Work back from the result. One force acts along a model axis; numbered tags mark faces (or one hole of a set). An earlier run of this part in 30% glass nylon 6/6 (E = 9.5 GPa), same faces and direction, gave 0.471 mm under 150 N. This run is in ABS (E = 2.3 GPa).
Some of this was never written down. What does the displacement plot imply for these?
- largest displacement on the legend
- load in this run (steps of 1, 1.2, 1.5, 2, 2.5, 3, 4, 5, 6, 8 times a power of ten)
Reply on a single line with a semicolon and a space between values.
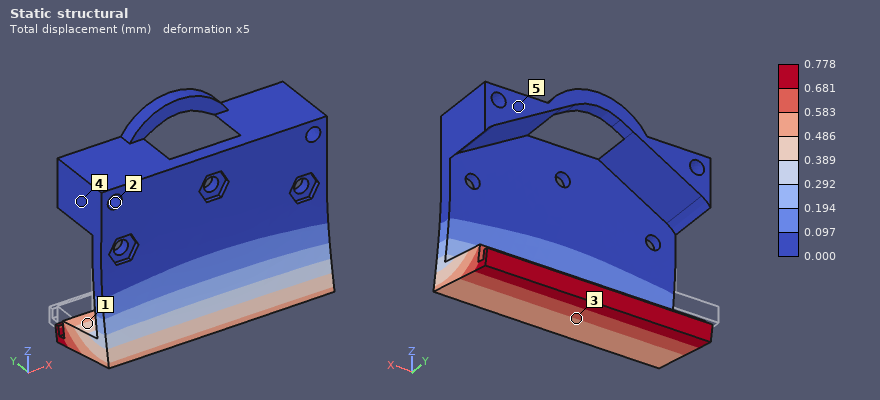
0.778 mm; 60 N
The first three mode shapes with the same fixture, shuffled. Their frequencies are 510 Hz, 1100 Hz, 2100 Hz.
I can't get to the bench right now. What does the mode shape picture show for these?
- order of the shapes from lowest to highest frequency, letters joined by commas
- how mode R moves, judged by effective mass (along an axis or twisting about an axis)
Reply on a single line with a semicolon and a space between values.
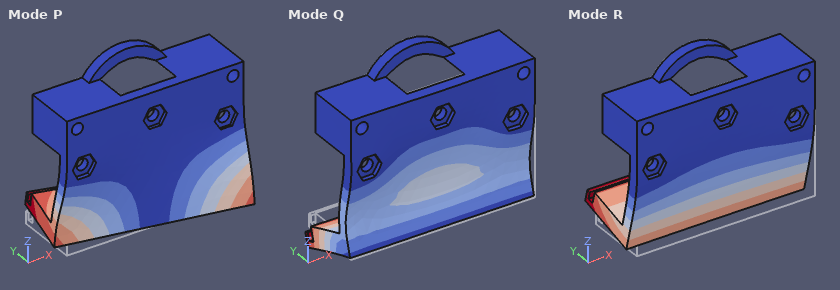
R, P, Q; along Y
